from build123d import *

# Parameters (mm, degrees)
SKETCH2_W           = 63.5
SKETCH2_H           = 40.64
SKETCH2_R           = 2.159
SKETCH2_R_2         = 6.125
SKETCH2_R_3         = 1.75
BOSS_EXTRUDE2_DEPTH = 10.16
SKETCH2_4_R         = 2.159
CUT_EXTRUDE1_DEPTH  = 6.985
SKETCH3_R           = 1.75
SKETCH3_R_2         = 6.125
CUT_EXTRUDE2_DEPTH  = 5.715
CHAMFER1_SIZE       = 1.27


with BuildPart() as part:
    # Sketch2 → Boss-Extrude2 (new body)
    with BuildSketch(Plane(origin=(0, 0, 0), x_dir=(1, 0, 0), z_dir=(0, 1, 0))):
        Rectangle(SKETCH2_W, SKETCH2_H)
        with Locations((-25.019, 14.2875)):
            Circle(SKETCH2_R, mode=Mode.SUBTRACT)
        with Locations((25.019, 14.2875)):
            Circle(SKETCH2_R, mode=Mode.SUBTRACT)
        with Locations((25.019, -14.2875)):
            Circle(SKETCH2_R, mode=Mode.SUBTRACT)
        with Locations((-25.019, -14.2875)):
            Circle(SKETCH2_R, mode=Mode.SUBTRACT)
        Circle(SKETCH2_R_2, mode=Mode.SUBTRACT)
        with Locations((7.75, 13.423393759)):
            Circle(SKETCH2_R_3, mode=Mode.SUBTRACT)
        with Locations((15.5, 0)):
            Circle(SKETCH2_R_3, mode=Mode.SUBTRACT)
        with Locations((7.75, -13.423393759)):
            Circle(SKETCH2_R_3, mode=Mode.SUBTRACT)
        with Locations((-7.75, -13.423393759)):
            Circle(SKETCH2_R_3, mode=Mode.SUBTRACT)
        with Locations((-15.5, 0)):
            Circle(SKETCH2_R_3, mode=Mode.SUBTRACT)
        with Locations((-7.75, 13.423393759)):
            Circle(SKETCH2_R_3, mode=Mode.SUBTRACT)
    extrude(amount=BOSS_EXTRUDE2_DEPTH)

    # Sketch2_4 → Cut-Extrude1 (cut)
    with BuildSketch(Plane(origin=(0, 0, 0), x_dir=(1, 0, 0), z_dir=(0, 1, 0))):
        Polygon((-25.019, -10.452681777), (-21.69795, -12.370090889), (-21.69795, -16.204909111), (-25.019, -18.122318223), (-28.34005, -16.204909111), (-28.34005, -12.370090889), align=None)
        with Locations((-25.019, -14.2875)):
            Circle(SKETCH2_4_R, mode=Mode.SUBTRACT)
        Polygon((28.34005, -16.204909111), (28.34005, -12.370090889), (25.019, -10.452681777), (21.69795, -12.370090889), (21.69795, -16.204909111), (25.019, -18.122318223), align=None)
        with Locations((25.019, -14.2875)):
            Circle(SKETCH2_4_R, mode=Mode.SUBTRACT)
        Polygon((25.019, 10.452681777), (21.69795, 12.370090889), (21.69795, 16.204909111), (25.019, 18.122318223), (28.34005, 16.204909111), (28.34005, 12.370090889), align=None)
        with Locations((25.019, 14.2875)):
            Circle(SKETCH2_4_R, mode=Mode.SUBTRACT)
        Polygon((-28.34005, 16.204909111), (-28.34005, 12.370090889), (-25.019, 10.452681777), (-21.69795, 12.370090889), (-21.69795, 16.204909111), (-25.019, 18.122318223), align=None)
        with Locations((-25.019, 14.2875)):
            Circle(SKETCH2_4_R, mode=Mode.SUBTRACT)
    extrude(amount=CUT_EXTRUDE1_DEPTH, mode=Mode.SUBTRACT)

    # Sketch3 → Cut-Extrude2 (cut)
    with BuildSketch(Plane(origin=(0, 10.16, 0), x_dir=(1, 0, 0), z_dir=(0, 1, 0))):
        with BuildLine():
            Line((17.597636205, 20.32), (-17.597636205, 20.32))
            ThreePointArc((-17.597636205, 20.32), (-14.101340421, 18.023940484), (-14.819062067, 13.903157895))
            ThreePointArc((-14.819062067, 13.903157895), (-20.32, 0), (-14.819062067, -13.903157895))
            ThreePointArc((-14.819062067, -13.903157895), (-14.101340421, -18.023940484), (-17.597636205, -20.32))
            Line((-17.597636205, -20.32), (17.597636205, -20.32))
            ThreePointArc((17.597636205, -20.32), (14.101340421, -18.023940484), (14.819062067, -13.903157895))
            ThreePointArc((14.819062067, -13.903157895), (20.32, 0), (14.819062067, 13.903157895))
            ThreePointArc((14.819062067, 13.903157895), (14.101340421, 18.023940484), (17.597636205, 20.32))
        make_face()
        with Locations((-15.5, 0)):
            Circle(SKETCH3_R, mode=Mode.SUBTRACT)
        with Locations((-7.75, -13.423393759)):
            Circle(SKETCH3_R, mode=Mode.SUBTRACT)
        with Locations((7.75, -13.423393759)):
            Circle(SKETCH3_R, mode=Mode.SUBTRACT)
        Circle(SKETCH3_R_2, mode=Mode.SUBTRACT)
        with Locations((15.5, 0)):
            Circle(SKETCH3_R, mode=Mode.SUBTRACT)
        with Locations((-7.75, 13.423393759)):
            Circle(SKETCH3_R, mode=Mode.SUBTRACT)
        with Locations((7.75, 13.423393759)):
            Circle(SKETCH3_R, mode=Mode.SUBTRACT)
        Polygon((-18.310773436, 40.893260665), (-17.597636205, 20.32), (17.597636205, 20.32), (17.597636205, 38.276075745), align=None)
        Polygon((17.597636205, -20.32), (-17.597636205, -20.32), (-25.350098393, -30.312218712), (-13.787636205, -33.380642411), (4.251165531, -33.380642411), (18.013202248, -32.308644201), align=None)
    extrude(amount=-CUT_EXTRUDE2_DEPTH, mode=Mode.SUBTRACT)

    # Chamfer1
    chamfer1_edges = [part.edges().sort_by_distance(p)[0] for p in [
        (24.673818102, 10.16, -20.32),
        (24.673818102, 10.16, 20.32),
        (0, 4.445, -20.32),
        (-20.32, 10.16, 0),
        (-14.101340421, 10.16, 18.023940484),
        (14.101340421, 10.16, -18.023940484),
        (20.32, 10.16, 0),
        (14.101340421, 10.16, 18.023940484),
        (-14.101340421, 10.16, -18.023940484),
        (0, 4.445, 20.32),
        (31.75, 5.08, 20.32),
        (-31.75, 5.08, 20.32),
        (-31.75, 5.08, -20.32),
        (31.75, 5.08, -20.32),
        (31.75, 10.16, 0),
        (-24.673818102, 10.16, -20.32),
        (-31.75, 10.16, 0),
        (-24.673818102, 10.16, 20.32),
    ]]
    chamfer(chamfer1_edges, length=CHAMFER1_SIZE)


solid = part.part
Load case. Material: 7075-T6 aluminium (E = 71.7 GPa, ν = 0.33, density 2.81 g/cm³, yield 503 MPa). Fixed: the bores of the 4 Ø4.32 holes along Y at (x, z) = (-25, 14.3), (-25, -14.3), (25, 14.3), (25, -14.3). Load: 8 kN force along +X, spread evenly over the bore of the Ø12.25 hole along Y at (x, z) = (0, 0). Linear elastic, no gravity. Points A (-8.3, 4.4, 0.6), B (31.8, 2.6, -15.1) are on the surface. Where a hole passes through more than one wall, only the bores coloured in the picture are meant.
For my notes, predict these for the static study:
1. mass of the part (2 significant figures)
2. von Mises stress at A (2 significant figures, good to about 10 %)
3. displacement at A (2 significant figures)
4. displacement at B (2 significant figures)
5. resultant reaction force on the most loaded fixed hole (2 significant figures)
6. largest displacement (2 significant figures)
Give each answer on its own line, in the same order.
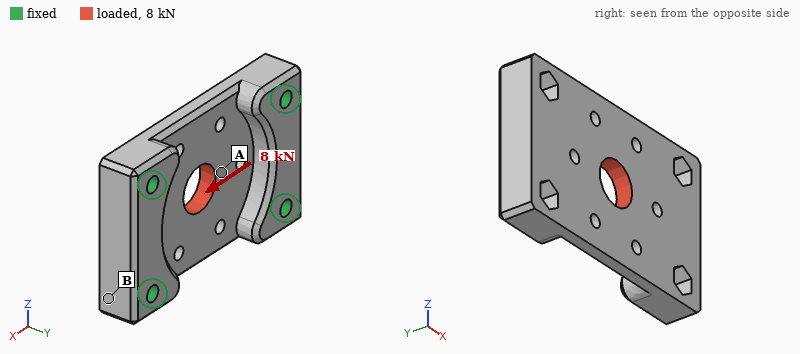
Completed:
45 g
49 MPa
32 µm
19 µm
2.0 kN
33 µm
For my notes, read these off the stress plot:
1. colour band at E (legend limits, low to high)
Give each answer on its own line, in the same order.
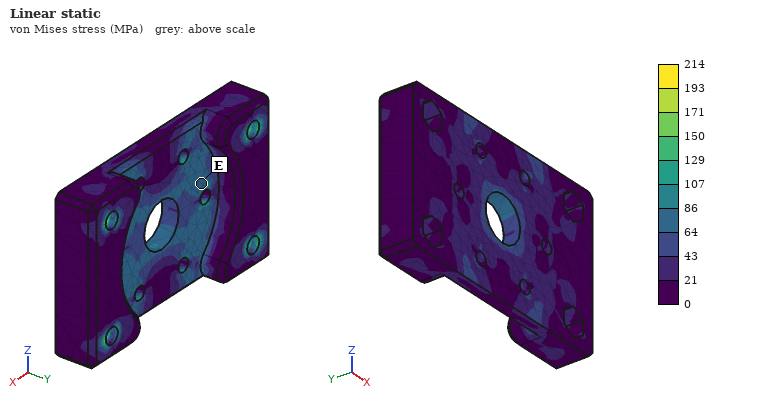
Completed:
64 to 86 MPa
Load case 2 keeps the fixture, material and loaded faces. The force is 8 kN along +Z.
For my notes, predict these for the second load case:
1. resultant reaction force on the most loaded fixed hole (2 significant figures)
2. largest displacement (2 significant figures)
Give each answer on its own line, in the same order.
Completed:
2.4 kN
34 µm
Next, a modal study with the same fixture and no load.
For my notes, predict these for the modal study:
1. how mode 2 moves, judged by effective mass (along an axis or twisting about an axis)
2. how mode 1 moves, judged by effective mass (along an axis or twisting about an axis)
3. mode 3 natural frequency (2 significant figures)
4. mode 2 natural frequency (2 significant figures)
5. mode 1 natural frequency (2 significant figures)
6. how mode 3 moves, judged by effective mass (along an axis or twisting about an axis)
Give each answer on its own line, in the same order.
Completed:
along X
along Y
16 kHz
14 kHz
12 kHz
twisting about X
